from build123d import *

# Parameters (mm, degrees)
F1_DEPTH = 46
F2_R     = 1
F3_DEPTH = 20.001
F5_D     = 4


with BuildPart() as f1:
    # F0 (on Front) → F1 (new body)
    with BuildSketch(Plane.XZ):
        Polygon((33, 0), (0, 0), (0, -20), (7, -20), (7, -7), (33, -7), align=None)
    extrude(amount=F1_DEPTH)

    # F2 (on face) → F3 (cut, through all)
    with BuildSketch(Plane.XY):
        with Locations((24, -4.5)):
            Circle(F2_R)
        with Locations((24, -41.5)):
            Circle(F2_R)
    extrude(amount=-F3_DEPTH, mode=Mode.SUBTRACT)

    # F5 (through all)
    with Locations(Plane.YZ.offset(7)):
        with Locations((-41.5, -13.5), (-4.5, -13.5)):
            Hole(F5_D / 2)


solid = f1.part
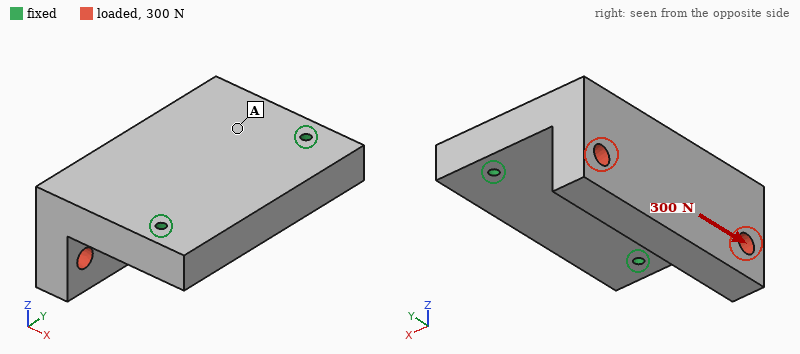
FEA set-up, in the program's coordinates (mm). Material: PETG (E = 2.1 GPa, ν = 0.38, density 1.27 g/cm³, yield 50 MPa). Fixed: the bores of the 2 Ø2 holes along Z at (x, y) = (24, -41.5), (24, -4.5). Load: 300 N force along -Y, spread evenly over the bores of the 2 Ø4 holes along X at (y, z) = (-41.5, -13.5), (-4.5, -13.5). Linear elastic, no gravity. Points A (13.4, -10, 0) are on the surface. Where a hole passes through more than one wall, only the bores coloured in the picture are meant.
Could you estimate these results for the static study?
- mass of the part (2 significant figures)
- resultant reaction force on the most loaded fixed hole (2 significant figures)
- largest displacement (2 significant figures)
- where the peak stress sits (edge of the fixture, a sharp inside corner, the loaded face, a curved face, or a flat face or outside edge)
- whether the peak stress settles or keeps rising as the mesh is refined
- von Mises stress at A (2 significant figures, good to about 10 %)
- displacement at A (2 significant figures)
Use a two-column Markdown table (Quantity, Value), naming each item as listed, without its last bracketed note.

| Quantity | Value |
|---|---|
| mass of the part | 19 g |
| resultant reaction force on the most loaded fixed hole | 240 N |
| largest displacement | 0.24 mm |
| where the peak stress sits | edge of the fixture |
| whether the peak stress settles or keeps rising as the mesh is refined | keeps rising |
| von Mises stress at A | 1.8 MPa |
| displacement at A | 0.050 mm |
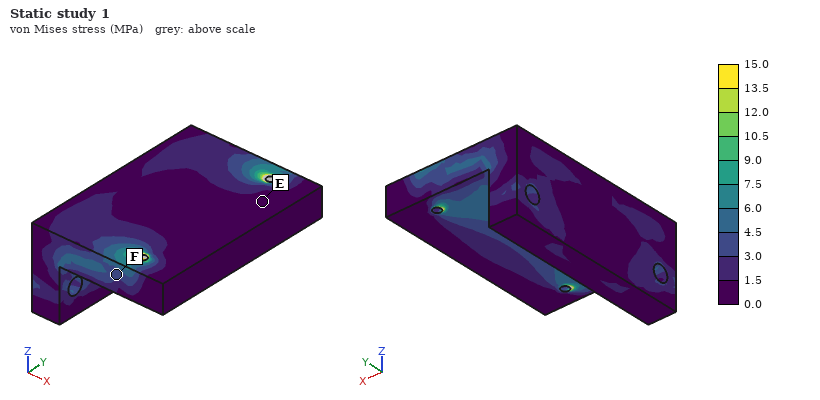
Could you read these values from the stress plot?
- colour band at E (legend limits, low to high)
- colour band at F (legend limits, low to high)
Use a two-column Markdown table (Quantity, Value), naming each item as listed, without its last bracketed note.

| Quantity | Value |
|---|---|
| colour band at E | 0.0 to 1.5 MPa |
| colour band at F | 3.0 to 4.5 MPa |
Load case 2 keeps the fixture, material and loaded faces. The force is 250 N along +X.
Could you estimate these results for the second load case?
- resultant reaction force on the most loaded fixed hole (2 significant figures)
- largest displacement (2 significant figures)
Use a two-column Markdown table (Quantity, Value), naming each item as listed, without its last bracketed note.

| Quantity | Value |
|---|---|
| resultant reaction force on the most loaded fixed hole | 130 N |
| largest displacement | 0.62 mm |
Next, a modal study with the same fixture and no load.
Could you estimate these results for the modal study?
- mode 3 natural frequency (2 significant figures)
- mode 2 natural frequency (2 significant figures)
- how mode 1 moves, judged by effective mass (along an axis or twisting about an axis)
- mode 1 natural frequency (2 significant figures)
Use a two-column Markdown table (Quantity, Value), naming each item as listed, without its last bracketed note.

| Quantity | Value |
|---|---|
| mode 3 natural frequency | 3500 Hz |
| mode 2 natural frequency | 2100 Hz |
| how mode 1 moves, judged by effective mass | along Z |
| mode 1 natural frequency | 1000 Hz |
